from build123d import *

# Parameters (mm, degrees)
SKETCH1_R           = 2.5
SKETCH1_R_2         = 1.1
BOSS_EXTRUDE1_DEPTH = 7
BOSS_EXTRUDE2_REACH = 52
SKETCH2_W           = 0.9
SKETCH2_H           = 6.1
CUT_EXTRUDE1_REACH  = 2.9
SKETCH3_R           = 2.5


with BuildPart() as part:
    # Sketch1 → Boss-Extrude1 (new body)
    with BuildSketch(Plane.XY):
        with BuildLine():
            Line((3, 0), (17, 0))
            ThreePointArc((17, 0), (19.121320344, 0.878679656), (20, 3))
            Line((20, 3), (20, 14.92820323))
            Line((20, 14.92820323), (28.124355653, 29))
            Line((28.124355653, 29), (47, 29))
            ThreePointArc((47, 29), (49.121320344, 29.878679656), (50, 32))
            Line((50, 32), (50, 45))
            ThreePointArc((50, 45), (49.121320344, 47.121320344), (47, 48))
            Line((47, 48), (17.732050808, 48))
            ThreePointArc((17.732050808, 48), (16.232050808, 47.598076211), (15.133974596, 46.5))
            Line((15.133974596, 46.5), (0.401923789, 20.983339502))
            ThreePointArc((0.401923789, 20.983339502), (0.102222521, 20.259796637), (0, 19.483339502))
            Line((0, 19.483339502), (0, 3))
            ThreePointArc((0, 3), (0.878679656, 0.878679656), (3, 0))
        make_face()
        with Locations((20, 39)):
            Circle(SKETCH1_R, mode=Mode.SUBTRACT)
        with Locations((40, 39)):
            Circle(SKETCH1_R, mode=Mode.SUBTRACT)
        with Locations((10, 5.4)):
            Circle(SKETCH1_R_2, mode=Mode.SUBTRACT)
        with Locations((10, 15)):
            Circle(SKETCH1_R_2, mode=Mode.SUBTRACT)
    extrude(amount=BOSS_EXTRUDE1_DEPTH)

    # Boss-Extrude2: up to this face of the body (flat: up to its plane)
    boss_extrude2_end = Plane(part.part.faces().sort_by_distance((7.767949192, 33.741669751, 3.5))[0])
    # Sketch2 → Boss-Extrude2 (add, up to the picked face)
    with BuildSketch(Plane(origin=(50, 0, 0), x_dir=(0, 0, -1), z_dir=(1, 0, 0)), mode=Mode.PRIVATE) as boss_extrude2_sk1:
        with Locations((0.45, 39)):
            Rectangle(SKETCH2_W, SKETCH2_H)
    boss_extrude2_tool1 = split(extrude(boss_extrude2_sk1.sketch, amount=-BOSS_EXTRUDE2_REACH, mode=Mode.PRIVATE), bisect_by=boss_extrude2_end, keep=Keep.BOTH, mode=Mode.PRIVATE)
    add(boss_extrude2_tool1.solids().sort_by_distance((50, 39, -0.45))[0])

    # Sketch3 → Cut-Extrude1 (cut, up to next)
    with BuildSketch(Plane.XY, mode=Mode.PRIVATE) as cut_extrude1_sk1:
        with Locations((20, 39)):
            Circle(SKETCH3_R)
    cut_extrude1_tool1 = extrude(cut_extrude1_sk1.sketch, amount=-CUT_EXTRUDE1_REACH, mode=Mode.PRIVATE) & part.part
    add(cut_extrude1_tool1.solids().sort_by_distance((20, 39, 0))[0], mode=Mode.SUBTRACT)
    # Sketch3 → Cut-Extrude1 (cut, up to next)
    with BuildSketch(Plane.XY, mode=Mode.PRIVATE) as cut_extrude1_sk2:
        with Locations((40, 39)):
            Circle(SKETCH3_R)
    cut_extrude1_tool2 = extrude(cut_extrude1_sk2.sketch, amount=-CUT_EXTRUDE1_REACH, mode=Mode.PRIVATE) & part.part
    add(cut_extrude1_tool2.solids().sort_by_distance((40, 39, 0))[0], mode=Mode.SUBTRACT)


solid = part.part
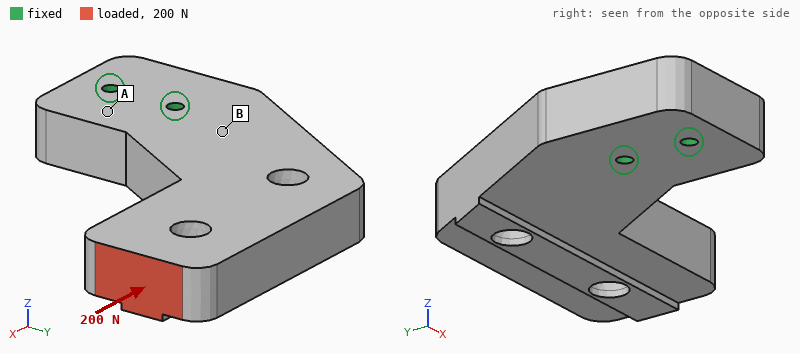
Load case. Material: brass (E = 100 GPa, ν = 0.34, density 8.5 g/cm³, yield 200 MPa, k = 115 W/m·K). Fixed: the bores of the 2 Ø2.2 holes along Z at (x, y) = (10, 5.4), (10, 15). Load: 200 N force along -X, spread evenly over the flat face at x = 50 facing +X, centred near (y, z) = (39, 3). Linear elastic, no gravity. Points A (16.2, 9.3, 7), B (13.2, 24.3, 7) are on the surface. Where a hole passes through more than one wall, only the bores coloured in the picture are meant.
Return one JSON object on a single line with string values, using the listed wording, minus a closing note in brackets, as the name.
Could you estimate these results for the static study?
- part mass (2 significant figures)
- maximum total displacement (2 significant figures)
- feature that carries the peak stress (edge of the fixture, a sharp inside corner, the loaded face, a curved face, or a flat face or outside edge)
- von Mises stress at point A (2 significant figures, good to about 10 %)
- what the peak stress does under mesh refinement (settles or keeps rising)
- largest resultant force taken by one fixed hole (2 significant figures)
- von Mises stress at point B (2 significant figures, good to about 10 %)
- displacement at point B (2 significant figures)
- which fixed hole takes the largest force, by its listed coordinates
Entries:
{"part mass": "79 g", "maximum total displacement": "15 µm", "feature that carries the peak stress": "edge of the fixture", "von Mises stress at point A": "7.2 MPa", "what the peak stress does under mesh refinement": "keeps rising", "largest resultant force taken by one fixed hole": "600 N", "von Mises stress at point B": "3.1 MPa", "displacement at point B": "2.3 µm", "which fixed hole takes the largest force, by its listed coordinates": "(10, 15)"}
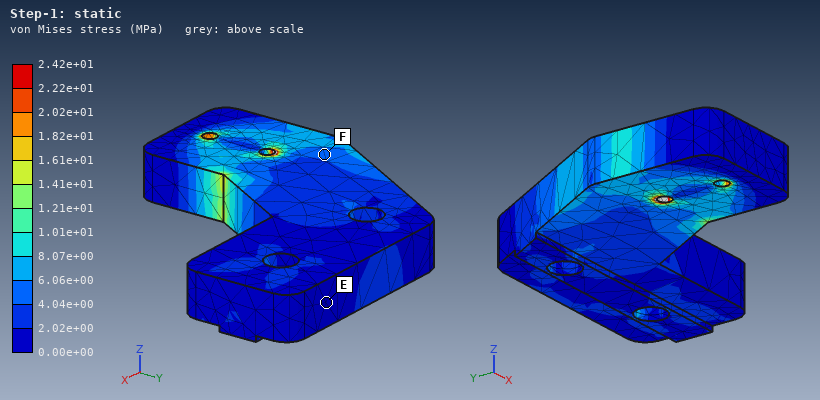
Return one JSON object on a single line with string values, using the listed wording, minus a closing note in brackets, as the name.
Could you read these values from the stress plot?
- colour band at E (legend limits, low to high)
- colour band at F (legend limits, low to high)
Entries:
{"colour band at E": "0.00e+00 to 2.02e+00 MPa", "colour band at F": "4.04e+00 to 6.06e+00 MPa"}
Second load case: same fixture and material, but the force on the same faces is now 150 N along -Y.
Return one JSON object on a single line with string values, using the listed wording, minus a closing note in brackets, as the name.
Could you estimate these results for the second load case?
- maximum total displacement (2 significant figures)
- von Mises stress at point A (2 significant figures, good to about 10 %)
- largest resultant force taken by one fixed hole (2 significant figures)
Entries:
{"maximum total displacement": "25 µm", "von Mises stress at point A": "9.7 MPa", "largest resultant force taken by one fixed hole": "520 N"}
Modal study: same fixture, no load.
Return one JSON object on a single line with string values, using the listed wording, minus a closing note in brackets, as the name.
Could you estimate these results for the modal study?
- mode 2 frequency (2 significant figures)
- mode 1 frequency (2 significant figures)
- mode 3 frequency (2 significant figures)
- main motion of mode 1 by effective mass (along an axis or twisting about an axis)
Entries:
{"mode 2 frequency": "2800 Hz", "mode 1 frequency": "1500 Hz", "mode 3 frequency": "4200 Hz", "main motion of mode 1 by effective mass": "along Z"}
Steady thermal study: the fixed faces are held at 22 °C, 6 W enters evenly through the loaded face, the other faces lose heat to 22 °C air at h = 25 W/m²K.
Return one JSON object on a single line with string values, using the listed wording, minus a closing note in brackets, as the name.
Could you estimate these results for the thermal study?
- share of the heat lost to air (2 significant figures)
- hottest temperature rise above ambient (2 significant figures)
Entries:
{"share of the heat lost to air": "13 %", "hottest temperature rise above ambient": "20 K"}
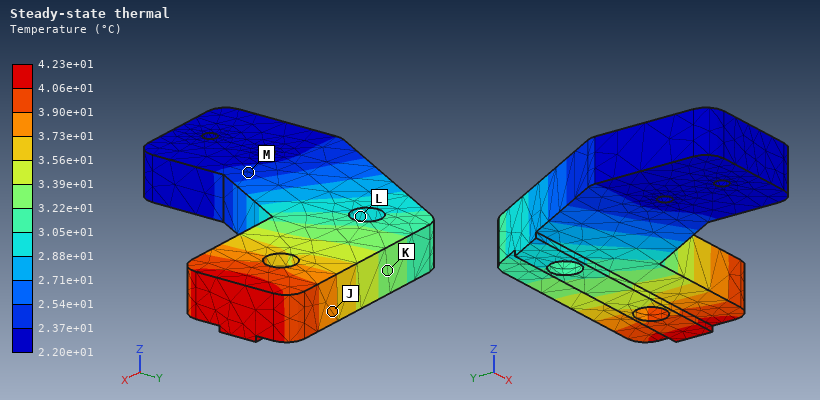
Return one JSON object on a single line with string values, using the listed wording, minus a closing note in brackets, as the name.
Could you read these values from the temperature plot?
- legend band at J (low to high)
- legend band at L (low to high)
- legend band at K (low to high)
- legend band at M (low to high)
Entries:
{"legend band at J": "3.73e+01 to 3.90e+01 °C", "legend band at L": "2.88e+01 to 3.05e+01 °C", "legend band at K": "3.22e+01 to 3.39e+01 °C", "legend band at M": "2.37e+01 to 2.54e+01 °C"}
